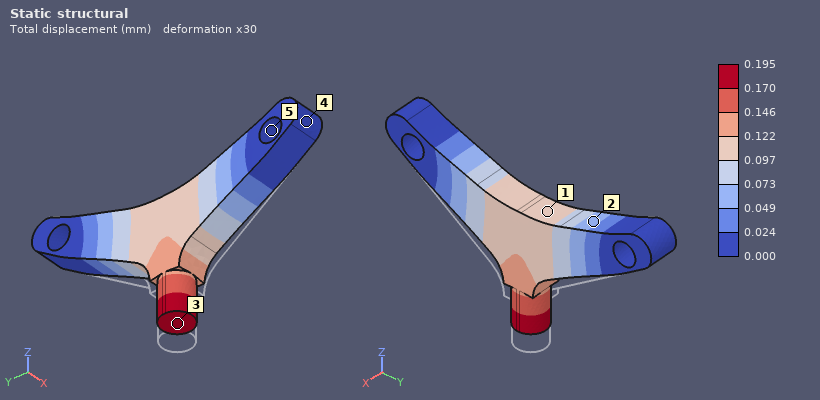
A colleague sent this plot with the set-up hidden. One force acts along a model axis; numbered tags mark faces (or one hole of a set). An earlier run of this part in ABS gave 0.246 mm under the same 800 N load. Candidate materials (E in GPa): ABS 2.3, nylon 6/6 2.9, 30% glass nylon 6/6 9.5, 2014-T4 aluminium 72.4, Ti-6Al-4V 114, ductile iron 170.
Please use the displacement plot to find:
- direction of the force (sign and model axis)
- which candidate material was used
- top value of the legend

+Z
nylon 6/6
0.195 mm
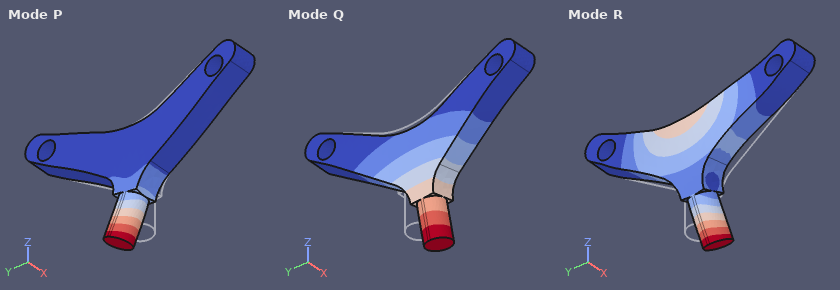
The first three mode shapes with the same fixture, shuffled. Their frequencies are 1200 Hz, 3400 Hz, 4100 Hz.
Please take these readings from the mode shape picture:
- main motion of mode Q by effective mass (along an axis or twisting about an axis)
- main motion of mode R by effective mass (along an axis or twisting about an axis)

along X
along X
